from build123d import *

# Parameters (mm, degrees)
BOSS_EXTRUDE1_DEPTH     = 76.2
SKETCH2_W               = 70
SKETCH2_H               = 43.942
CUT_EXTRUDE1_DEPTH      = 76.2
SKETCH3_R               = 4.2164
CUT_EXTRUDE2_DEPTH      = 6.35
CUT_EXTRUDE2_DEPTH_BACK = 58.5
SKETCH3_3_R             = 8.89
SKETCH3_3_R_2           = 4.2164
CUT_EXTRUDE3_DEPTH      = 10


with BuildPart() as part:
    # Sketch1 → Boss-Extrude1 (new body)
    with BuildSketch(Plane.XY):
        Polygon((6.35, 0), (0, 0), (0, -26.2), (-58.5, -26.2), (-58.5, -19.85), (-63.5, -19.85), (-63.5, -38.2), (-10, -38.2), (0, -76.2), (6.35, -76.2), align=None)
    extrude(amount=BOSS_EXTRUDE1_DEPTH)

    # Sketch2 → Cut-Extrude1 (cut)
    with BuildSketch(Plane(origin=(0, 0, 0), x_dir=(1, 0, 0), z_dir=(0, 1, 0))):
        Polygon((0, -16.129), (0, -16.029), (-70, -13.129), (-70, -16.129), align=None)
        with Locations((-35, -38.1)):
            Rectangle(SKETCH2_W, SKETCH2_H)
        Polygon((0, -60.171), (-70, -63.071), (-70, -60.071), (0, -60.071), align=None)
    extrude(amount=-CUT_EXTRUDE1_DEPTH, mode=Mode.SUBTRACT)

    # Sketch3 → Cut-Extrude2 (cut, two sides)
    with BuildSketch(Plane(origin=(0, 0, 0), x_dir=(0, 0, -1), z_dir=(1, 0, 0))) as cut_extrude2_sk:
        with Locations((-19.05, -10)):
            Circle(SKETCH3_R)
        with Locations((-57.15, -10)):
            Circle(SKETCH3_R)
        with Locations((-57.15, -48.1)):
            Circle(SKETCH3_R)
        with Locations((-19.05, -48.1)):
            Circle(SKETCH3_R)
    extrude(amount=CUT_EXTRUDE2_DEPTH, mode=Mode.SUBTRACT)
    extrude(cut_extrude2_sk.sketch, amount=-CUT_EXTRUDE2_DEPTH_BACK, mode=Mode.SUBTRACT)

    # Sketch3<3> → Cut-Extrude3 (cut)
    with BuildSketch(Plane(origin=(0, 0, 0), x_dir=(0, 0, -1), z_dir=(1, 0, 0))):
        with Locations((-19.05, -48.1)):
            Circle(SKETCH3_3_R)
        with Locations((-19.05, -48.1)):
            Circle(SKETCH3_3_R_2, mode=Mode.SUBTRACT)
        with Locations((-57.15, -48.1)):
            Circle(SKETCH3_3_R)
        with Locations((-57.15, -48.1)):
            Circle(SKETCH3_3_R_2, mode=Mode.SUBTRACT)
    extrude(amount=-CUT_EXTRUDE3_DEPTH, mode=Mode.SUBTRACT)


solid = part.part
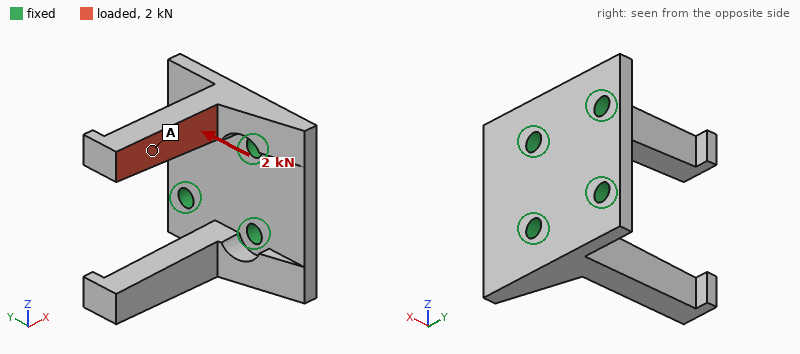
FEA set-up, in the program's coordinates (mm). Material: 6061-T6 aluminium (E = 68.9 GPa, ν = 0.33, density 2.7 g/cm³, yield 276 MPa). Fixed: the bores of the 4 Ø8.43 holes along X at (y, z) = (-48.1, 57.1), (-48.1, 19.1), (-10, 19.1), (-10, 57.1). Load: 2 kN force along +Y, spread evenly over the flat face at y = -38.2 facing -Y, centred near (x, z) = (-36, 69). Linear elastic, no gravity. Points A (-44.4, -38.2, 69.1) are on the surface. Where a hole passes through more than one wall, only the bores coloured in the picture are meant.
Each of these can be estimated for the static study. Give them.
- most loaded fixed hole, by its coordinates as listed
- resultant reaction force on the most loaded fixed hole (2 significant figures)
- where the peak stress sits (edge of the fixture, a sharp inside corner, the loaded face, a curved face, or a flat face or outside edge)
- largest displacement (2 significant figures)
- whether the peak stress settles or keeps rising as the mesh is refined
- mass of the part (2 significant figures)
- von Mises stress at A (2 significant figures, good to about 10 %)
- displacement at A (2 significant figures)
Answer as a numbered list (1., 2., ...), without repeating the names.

1. (-48.1, 57.1)
2. 2.7 kN
3. edge of the fixture
4. 0.57 mm
5. keeps rising
6. 170 g
7. 20 MPa
8. 0.34 mm
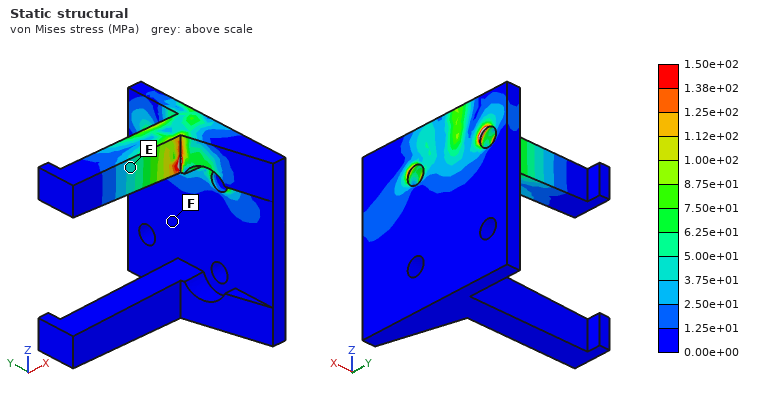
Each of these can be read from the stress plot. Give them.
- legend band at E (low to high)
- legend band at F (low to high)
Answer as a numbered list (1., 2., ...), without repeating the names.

1. 3.75e+01 to 5.00e+01 MPa
2. 0.00e+00 to 1.25e+01 MPa
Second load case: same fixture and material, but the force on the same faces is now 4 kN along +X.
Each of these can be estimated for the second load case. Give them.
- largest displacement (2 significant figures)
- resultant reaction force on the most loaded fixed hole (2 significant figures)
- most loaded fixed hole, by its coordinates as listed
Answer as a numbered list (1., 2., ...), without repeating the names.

1. 0.27 mm
2. 3.2 kN
3. (-48.1, 57.1)
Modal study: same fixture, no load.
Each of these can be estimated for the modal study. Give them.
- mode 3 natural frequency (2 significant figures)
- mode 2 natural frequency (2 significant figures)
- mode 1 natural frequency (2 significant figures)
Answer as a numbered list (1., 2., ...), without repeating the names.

1. 2200 Hz
2. 1800 Hz
3. 1800 Hz
